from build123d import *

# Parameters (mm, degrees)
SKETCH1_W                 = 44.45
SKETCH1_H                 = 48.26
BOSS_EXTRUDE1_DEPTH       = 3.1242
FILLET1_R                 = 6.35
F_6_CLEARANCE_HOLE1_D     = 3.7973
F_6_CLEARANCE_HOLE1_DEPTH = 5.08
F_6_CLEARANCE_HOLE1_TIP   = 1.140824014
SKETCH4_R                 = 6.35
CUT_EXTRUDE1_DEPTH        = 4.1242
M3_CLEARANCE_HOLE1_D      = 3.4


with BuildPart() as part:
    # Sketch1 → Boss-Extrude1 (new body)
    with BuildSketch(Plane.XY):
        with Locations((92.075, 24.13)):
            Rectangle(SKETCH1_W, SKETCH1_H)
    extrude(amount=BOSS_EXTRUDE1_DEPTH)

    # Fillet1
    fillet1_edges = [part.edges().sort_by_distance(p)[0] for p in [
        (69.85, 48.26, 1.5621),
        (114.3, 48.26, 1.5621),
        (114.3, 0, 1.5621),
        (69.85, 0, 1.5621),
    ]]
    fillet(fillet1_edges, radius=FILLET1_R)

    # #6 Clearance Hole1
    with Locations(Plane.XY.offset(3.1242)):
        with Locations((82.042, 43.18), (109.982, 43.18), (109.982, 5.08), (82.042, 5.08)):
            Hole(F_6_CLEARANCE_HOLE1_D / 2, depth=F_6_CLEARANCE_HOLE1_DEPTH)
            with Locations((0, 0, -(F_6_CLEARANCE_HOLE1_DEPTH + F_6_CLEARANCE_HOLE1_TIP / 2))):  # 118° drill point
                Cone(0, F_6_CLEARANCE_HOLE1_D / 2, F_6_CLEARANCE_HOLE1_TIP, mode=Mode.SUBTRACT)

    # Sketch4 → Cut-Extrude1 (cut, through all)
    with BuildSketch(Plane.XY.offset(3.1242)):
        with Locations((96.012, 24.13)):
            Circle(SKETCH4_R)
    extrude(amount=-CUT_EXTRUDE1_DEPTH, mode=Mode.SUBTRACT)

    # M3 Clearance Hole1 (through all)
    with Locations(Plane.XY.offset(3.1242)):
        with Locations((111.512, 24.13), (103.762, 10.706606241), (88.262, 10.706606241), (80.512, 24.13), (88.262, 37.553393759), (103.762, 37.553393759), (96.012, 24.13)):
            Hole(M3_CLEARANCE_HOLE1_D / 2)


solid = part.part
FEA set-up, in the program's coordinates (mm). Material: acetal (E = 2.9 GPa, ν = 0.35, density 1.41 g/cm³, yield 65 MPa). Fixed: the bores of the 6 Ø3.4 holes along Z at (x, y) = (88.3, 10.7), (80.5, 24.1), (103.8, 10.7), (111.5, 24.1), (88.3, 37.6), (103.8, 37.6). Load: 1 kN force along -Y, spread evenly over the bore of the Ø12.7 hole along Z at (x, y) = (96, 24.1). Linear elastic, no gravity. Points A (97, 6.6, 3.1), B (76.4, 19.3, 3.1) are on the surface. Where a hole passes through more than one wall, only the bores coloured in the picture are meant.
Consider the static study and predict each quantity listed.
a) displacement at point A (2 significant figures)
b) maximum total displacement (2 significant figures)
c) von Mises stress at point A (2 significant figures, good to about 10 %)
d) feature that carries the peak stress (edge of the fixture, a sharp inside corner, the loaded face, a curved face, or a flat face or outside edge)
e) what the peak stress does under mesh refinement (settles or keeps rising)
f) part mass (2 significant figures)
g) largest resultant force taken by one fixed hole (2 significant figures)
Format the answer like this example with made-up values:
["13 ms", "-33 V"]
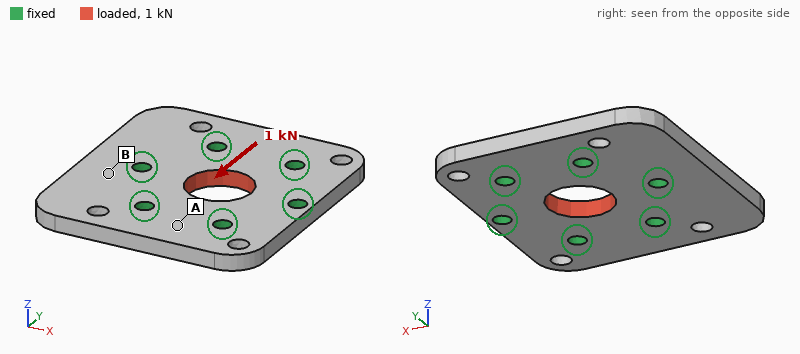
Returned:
["9.9 µm", "30 µm", "2.3 MPa", "edge of the fixture", "keeps rising", "8.3 g", "220 N"]
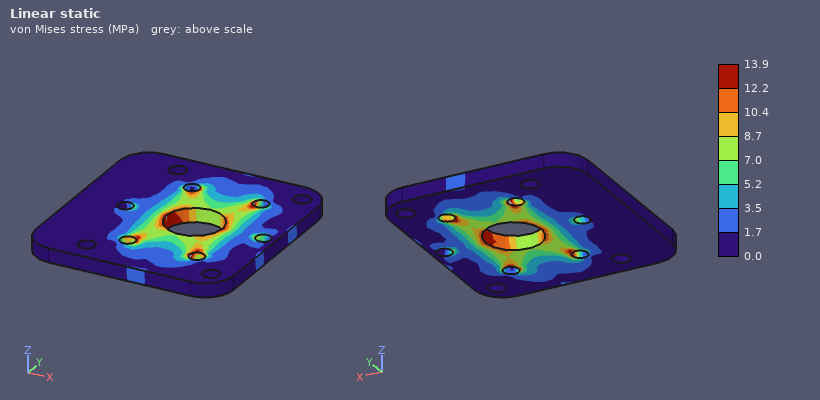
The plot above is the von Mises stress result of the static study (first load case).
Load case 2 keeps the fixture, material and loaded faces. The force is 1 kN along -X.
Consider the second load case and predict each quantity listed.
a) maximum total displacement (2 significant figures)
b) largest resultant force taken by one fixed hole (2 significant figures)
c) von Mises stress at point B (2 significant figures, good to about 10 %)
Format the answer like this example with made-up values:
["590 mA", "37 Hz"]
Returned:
["29 µm", "250 N", "1.8 MPa"]
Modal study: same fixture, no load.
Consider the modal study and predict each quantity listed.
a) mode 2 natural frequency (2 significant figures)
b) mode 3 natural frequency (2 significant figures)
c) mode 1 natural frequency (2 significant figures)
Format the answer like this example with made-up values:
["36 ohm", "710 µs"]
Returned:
["3000 Hz", "5900 Hz", "2900 Hz"]
